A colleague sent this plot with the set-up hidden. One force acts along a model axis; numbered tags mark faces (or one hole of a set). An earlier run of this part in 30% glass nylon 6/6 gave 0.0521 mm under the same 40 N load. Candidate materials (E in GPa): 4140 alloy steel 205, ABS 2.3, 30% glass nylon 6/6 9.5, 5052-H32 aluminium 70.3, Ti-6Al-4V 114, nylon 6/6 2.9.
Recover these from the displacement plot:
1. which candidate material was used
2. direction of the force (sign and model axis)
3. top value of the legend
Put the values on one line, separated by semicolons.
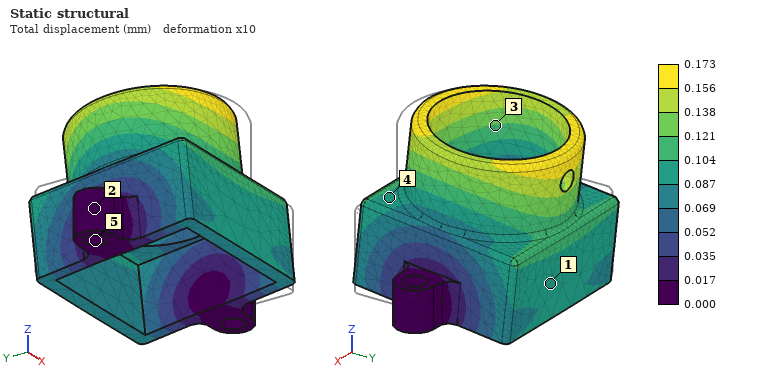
nylon 6/6; +Y; 0.173 mm
